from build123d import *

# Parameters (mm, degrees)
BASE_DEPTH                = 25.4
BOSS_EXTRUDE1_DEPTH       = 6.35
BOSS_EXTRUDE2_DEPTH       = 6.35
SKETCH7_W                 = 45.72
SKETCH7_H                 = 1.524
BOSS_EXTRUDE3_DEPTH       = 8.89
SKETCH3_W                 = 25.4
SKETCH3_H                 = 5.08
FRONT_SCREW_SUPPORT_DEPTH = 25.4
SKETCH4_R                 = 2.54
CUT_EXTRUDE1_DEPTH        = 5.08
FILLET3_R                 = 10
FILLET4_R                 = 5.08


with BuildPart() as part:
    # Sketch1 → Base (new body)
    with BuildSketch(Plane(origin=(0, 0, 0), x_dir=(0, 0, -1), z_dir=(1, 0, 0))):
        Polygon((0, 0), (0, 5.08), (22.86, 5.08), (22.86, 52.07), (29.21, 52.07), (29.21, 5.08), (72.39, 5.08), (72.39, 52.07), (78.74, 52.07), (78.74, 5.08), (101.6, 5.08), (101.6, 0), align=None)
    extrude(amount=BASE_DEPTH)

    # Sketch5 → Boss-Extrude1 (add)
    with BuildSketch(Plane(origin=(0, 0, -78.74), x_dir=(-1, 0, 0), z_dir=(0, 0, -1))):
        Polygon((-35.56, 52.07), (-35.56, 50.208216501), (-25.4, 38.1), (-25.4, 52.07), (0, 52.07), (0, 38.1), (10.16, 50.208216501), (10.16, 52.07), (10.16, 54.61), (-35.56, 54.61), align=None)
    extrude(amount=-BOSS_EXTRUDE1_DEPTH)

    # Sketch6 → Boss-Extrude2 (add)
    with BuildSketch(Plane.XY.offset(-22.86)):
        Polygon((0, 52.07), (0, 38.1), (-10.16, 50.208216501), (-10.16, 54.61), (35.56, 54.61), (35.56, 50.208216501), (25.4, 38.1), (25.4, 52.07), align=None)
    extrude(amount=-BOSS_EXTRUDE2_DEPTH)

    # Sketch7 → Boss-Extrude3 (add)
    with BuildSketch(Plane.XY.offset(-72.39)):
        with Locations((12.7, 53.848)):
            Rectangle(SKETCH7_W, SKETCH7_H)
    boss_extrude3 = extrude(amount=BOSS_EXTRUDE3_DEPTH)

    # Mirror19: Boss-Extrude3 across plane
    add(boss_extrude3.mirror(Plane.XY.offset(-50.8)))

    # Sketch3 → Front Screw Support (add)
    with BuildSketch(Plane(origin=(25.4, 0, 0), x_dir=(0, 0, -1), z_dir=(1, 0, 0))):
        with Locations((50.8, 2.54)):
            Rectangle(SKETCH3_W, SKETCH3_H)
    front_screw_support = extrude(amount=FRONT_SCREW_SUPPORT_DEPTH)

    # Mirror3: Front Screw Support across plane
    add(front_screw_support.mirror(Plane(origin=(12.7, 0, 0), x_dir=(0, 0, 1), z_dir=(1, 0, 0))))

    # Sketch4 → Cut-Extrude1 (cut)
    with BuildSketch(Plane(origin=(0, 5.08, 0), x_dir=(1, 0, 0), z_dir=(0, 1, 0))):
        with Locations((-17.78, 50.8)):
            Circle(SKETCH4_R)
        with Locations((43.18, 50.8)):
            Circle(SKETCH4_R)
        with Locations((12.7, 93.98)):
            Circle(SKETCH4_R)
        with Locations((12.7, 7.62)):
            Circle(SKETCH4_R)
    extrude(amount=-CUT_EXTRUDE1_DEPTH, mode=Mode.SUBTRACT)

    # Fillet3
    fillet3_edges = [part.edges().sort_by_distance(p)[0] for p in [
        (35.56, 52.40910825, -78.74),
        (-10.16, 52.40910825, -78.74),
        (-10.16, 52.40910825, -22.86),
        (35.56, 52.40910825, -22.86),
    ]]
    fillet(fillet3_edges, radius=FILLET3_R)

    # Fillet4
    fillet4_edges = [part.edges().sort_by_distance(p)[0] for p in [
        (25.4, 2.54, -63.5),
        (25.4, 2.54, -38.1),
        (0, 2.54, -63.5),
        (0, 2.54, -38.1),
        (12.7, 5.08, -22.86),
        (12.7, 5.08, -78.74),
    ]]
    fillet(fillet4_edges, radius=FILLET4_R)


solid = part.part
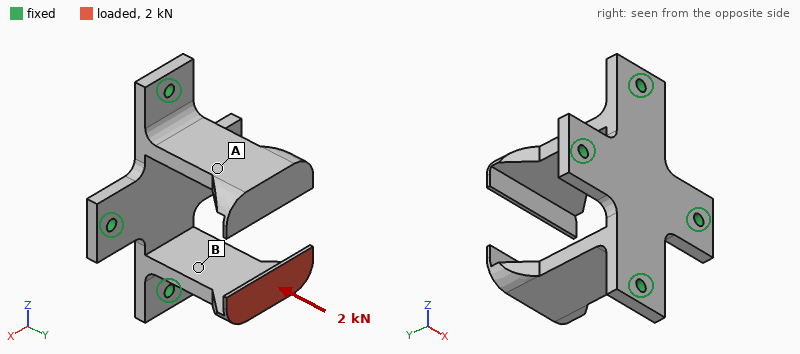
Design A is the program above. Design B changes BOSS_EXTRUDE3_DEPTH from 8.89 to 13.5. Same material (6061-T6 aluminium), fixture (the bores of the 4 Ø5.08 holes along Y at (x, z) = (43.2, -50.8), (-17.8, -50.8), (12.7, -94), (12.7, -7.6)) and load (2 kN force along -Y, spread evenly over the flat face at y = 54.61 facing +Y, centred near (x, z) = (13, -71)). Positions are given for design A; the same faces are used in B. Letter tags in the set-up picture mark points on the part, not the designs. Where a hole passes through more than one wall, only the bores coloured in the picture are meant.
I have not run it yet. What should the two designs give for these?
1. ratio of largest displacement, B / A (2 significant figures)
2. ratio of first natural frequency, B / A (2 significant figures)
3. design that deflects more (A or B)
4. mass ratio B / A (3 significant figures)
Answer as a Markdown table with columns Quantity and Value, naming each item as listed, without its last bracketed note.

| Quantity | Value |
|---|---|
| ratio of largest displacement, B / A | 1.8 |
| ratio of first natural frequency, B / A | 0.95 |
| design that deflects more | B |
| mass ratio B / A | 1.02 |
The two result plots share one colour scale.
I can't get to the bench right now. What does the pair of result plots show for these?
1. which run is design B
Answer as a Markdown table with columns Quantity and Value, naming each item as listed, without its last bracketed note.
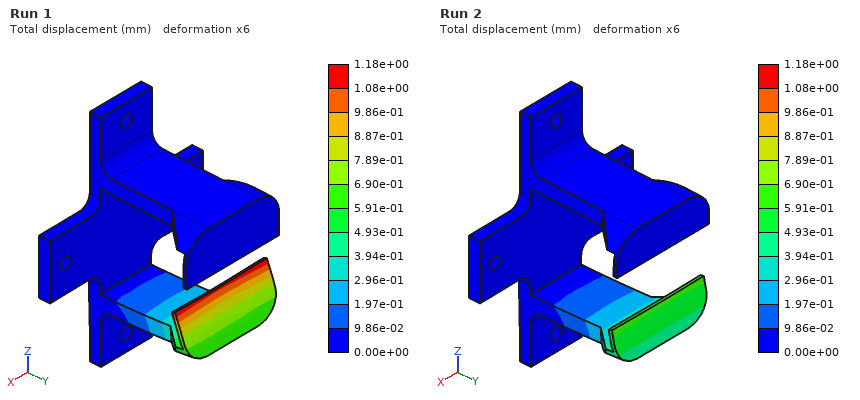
| Quantity | Value |
|---|---|
| which run is design B | Run 1 |
